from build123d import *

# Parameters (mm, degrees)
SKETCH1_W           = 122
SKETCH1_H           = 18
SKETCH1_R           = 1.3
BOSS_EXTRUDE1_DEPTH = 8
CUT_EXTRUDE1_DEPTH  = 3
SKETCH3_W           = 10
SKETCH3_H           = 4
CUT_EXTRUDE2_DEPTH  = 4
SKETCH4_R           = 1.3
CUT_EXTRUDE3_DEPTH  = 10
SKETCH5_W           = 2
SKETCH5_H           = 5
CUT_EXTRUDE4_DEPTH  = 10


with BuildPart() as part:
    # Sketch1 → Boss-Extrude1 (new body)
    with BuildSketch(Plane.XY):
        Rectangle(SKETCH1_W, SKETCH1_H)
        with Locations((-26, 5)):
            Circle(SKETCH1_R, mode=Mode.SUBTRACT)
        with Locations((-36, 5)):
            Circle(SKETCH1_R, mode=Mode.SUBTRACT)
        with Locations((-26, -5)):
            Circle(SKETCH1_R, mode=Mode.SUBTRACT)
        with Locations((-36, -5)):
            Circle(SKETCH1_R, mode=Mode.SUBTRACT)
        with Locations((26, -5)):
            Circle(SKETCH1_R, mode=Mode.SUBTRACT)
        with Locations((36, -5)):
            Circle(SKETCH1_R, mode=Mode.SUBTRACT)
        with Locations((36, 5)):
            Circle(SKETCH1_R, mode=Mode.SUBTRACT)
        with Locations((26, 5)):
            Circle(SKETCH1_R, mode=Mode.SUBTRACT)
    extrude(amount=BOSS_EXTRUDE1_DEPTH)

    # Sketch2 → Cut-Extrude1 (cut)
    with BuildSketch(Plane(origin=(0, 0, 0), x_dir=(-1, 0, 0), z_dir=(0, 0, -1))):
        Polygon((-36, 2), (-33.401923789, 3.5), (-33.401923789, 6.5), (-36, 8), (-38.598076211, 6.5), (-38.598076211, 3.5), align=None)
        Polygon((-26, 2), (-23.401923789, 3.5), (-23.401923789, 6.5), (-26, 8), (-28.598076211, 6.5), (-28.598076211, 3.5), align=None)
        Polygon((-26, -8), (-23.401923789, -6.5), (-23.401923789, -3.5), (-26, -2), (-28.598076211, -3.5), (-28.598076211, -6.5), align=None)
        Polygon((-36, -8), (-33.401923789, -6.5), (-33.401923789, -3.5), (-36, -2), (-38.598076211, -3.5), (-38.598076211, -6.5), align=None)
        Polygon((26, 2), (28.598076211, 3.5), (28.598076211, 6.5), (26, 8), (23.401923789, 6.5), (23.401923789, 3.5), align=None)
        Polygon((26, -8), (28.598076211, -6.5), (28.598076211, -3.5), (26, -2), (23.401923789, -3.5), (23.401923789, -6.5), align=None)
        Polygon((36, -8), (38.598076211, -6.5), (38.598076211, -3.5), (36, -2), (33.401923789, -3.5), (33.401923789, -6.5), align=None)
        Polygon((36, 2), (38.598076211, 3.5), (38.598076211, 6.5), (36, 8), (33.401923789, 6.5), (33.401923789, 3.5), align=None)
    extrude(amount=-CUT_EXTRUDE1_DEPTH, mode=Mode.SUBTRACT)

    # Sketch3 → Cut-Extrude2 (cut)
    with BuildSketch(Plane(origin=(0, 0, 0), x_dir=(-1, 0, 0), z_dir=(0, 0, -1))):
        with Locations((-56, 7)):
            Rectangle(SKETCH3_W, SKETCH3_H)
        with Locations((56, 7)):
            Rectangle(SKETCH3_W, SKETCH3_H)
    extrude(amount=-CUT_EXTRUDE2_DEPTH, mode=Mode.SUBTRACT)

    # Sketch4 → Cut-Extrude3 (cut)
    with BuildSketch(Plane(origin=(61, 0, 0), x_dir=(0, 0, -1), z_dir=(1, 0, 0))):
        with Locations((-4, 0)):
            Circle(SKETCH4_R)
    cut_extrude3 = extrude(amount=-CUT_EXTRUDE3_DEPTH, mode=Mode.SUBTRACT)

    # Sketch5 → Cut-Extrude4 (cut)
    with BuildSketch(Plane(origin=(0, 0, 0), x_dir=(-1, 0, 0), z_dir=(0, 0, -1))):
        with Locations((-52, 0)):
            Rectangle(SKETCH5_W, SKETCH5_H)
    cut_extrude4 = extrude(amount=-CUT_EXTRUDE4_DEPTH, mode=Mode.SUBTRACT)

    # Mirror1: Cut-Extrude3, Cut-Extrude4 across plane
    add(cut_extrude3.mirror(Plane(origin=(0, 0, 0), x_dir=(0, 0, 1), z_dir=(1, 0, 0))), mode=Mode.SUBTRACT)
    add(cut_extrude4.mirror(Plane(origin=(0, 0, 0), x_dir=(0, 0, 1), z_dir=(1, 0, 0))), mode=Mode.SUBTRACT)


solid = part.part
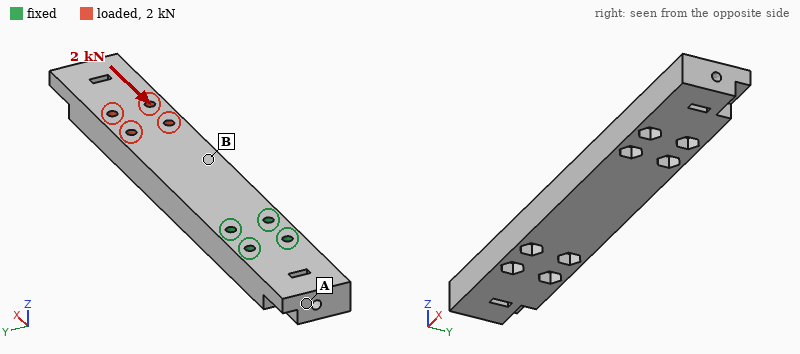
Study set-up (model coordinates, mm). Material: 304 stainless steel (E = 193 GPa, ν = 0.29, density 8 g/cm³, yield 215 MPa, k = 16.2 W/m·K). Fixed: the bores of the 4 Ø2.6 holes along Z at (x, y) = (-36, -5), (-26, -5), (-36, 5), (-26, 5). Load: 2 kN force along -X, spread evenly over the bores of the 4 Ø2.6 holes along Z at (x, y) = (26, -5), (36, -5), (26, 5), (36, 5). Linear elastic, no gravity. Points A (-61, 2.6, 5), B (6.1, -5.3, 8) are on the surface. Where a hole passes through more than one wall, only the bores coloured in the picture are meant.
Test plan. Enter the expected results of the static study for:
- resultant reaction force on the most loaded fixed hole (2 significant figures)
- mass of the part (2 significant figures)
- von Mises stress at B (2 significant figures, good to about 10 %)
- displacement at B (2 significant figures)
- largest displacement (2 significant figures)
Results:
880 N
130 g
30 MPa
11 µm
65 µm
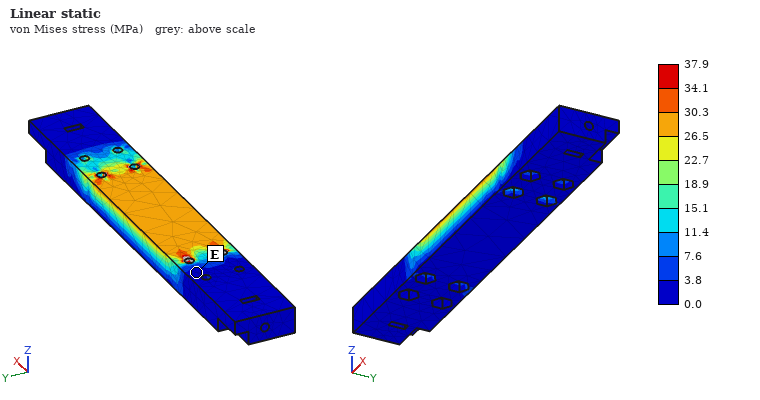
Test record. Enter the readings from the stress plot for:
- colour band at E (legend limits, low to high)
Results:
0.0 to 3.8 MPa
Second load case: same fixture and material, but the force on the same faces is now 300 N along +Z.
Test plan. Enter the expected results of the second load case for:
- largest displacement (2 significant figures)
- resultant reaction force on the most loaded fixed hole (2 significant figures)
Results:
0.27 mm
640 N
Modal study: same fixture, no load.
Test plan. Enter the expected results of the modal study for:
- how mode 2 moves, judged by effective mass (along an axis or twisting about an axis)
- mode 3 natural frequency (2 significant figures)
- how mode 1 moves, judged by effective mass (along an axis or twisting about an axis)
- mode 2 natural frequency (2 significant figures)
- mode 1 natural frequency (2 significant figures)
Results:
along Y
4500 Hz
along Z
1800 Hz
800 Hz
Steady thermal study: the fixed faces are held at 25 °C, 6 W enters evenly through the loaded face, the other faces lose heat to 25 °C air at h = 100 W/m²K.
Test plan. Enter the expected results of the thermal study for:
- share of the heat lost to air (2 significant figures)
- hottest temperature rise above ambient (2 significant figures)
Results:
94 %
26 K
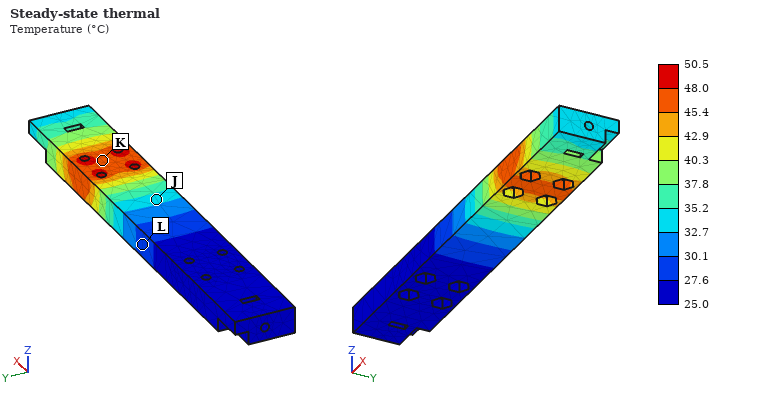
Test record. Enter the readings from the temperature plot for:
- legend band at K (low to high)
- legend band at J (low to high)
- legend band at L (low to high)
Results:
45.4 to 48.0 °C
32.7 to 35.2 °C
27.6 to 30.1 °C
